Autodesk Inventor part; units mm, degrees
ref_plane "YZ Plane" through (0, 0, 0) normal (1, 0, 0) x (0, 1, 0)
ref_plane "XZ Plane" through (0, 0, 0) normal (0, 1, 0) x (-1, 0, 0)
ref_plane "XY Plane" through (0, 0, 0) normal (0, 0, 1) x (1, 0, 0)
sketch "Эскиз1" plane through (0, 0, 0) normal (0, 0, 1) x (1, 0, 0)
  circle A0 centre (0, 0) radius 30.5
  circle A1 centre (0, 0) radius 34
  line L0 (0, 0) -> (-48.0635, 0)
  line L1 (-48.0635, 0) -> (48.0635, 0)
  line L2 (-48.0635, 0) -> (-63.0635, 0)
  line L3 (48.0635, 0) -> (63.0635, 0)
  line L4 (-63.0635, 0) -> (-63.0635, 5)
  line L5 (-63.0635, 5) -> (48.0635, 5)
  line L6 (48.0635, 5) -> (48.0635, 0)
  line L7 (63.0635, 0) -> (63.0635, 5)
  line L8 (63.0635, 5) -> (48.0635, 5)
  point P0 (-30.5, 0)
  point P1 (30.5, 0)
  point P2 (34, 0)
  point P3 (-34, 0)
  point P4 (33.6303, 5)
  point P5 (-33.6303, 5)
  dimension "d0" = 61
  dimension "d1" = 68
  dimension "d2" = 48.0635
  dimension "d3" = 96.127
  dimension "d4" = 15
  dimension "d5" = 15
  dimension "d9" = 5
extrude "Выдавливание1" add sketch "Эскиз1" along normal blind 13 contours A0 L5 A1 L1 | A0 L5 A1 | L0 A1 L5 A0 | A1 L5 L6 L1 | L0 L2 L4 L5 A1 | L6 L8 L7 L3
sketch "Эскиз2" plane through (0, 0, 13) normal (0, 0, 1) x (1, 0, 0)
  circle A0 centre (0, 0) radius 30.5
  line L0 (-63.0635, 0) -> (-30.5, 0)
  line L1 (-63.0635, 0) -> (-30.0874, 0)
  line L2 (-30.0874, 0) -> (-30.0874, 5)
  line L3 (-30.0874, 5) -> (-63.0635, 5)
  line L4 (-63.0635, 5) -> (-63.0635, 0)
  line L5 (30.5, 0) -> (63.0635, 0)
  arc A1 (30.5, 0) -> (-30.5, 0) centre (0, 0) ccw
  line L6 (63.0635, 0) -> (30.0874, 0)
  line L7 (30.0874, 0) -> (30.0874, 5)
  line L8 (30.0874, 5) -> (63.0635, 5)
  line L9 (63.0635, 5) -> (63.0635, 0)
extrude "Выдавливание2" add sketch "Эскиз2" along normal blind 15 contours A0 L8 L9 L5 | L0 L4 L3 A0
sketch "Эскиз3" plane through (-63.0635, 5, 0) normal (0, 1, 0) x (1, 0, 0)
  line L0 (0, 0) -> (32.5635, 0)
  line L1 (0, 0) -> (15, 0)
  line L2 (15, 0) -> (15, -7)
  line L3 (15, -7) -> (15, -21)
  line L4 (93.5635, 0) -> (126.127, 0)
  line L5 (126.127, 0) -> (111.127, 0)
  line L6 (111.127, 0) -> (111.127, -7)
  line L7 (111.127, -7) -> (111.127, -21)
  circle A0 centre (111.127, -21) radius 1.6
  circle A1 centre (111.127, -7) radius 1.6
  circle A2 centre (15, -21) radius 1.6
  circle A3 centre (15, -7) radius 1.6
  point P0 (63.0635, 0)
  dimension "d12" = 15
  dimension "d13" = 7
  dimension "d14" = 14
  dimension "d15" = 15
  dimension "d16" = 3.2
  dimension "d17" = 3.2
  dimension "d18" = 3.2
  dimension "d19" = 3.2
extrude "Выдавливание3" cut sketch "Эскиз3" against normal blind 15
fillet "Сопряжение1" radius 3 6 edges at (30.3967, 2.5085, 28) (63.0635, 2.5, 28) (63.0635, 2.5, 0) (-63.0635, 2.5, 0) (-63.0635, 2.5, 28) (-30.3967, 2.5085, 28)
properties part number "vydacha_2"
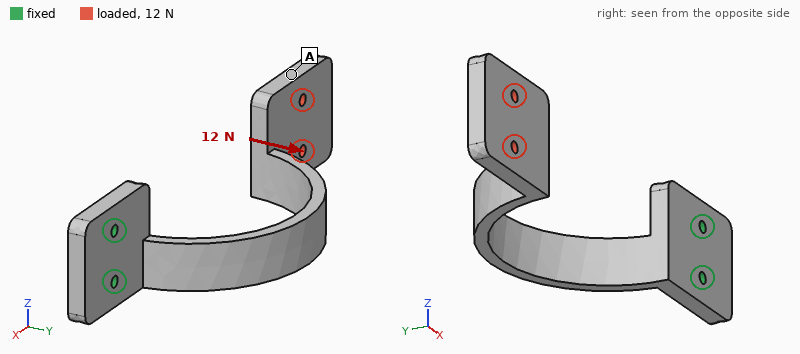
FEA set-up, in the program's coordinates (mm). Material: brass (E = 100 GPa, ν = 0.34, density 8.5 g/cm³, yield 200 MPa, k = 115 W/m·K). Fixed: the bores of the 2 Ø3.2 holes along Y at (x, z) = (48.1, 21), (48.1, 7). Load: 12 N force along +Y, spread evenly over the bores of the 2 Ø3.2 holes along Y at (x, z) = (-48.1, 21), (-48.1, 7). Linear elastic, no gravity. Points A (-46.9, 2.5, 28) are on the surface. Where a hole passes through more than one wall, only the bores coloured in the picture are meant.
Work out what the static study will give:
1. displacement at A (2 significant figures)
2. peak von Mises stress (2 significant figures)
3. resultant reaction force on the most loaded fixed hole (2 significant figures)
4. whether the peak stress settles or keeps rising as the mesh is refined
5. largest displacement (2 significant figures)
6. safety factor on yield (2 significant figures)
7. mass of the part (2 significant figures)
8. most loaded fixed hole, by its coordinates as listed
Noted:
0.77 mm
42 MPa
8.1 N
settles
0.97 mm
4.8
110 g
(48.1, 21)
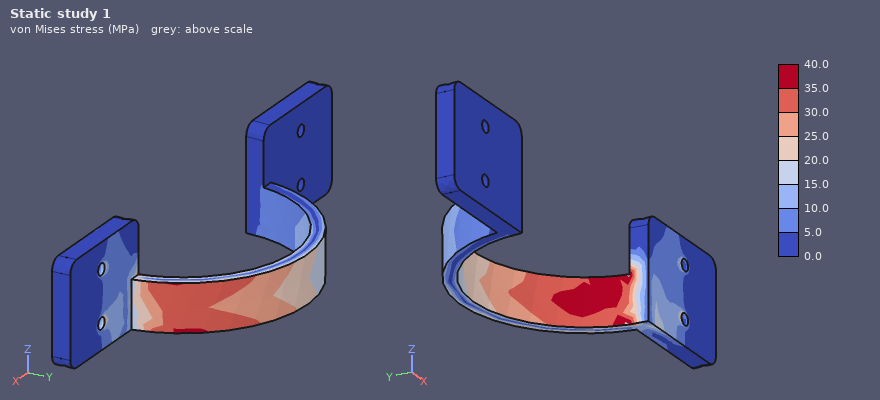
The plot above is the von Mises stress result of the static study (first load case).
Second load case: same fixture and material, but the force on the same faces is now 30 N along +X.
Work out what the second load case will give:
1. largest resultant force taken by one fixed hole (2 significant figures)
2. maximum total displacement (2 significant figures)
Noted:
16 N
0.82 mm
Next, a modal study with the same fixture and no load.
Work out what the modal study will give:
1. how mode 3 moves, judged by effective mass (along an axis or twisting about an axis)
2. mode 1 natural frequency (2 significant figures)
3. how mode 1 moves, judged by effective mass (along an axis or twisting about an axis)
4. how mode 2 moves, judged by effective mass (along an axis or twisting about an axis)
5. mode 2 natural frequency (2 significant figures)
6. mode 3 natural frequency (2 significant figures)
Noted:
along X
94 Hz
along Y
along Z
140 Hz
360 Hz
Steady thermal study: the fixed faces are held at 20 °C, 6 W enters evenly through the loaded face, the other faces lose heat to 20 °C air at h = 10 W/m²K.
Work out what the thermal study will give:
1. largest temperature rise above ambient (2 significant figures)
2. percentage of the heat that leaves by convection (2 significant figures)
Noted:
76 K
47 %
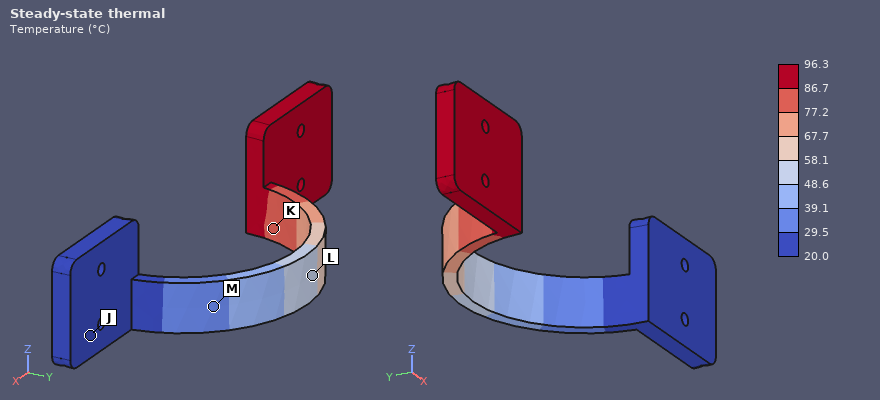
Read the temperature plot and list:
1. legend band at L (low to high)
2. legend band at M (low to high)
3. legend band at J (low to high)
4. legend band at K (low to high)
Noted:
48.6 to 58.1 °C
29.5 to 39.1 °C
20.0 to 29.5 °C
77.2 to 86.7 °C
